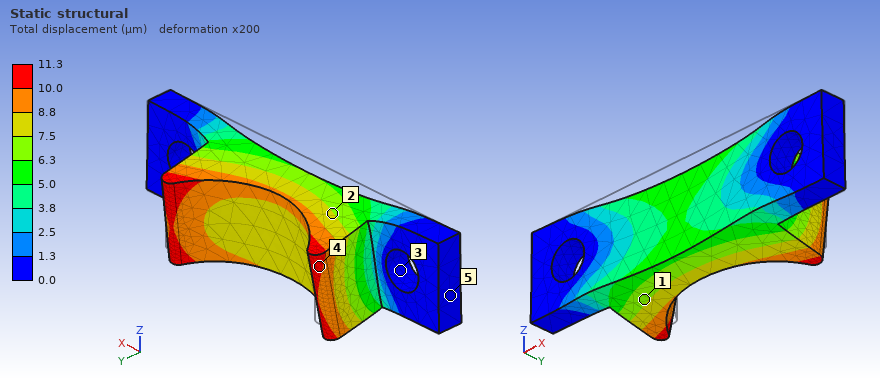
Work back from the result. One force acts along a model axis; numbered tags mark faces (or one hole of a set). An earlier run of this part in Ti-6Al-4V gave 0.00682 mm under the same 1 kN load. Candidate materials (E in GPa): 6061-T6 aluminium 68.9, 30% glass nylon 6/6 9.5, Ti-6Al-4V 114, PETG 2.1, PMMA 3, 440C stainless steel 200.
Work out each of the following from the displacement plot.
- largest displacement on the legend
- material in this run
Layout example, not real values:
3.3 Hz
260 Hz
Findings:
11.3 µm
6061-T6 aluminium
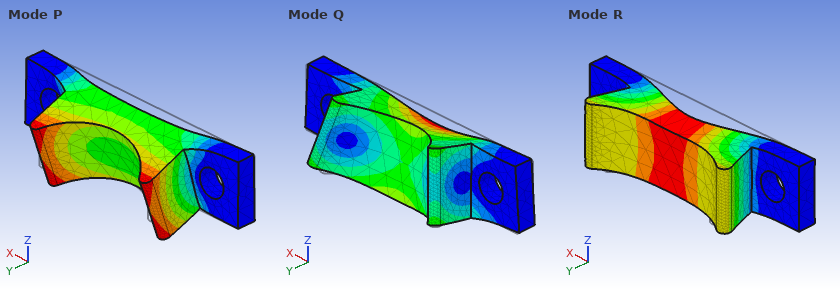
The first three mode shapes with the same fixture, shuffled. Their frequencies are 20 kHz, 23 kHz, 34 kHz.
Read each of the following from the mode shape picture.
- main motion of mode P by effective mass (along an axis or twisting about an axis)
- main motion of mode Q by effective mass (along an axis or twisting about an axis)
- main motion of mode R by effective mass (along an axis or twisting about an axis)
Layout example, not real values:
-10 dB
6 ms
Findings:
along Z
along Z
along Y
